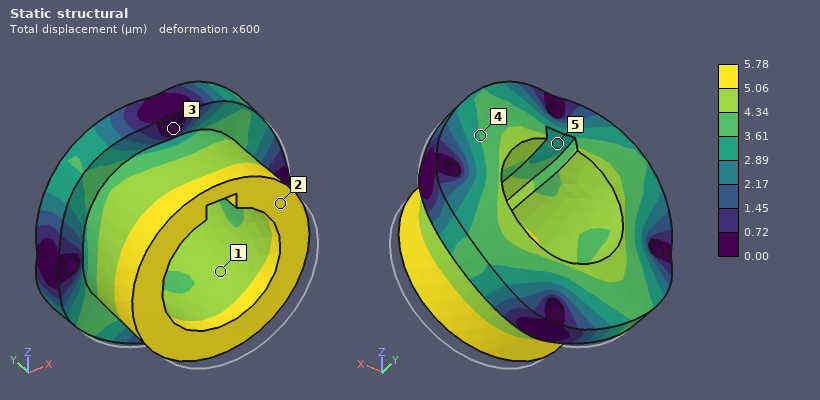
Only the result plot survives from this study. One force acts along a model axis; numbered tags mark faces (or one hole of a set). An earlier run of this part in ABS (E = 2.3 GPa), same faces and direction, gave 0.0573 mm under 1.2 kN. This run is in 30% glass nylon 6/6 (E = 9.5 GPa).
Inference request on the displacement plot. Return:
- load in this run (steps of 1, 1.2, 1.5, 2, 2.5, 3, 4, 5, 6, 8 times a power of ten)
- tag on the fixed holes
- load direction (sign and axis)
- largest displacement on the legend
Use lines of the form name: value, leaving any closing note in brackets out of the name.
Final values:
load in this run: 500 N
tag on the fixed holes: 3
load direction: +Y
largest displacement on the legend: 5.78 µm
